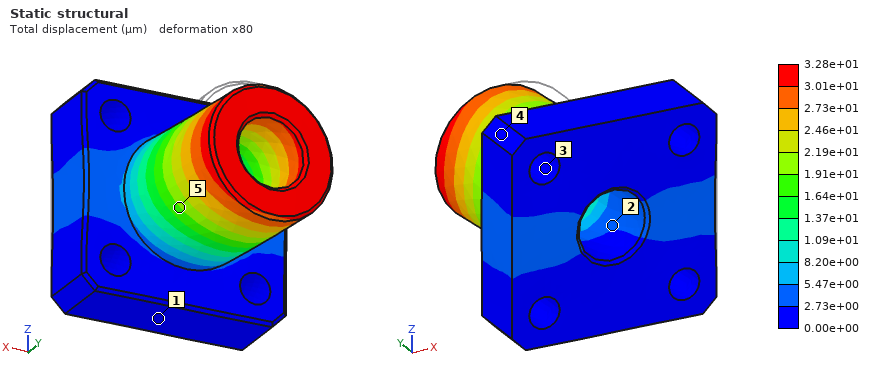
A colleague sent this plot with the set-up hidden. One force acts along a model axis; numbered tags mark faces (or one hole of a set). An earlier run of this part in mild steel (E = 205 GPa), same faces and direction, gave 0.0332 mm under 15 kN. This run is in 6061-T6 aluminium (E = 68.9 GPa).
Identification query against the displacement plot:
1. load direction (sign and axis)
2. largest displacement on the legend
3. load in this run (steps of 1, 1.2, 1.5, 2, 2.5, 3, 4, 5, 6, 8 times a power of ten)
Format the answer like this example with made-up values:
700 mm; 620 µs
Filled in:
-X; 3.28e+01 µm; 5 kN
